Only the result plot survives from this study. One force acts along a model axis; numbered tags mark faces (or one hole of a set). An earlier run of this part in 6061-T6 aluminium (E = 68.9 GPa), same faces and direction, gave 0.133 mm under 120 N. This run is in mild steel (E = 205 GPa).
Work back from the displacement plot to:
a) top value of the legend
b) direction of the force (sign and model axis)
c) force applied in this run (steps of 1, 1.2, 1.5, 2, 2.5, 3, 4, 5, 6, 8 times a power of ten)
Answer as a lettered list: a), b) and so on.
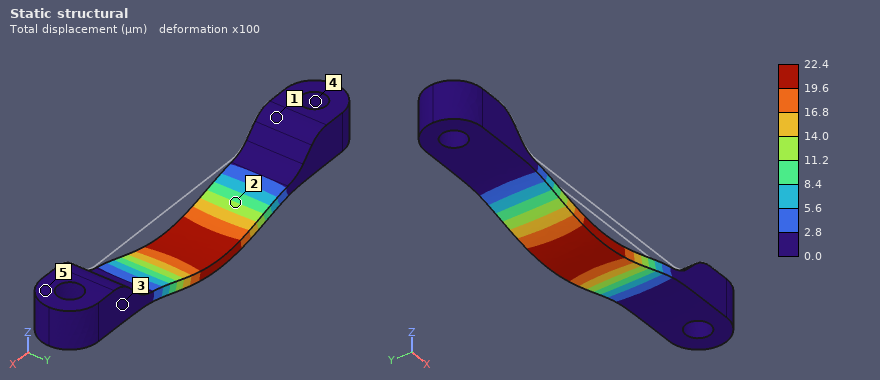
a) 22.4 µm
b) -Z
c) 60 N
